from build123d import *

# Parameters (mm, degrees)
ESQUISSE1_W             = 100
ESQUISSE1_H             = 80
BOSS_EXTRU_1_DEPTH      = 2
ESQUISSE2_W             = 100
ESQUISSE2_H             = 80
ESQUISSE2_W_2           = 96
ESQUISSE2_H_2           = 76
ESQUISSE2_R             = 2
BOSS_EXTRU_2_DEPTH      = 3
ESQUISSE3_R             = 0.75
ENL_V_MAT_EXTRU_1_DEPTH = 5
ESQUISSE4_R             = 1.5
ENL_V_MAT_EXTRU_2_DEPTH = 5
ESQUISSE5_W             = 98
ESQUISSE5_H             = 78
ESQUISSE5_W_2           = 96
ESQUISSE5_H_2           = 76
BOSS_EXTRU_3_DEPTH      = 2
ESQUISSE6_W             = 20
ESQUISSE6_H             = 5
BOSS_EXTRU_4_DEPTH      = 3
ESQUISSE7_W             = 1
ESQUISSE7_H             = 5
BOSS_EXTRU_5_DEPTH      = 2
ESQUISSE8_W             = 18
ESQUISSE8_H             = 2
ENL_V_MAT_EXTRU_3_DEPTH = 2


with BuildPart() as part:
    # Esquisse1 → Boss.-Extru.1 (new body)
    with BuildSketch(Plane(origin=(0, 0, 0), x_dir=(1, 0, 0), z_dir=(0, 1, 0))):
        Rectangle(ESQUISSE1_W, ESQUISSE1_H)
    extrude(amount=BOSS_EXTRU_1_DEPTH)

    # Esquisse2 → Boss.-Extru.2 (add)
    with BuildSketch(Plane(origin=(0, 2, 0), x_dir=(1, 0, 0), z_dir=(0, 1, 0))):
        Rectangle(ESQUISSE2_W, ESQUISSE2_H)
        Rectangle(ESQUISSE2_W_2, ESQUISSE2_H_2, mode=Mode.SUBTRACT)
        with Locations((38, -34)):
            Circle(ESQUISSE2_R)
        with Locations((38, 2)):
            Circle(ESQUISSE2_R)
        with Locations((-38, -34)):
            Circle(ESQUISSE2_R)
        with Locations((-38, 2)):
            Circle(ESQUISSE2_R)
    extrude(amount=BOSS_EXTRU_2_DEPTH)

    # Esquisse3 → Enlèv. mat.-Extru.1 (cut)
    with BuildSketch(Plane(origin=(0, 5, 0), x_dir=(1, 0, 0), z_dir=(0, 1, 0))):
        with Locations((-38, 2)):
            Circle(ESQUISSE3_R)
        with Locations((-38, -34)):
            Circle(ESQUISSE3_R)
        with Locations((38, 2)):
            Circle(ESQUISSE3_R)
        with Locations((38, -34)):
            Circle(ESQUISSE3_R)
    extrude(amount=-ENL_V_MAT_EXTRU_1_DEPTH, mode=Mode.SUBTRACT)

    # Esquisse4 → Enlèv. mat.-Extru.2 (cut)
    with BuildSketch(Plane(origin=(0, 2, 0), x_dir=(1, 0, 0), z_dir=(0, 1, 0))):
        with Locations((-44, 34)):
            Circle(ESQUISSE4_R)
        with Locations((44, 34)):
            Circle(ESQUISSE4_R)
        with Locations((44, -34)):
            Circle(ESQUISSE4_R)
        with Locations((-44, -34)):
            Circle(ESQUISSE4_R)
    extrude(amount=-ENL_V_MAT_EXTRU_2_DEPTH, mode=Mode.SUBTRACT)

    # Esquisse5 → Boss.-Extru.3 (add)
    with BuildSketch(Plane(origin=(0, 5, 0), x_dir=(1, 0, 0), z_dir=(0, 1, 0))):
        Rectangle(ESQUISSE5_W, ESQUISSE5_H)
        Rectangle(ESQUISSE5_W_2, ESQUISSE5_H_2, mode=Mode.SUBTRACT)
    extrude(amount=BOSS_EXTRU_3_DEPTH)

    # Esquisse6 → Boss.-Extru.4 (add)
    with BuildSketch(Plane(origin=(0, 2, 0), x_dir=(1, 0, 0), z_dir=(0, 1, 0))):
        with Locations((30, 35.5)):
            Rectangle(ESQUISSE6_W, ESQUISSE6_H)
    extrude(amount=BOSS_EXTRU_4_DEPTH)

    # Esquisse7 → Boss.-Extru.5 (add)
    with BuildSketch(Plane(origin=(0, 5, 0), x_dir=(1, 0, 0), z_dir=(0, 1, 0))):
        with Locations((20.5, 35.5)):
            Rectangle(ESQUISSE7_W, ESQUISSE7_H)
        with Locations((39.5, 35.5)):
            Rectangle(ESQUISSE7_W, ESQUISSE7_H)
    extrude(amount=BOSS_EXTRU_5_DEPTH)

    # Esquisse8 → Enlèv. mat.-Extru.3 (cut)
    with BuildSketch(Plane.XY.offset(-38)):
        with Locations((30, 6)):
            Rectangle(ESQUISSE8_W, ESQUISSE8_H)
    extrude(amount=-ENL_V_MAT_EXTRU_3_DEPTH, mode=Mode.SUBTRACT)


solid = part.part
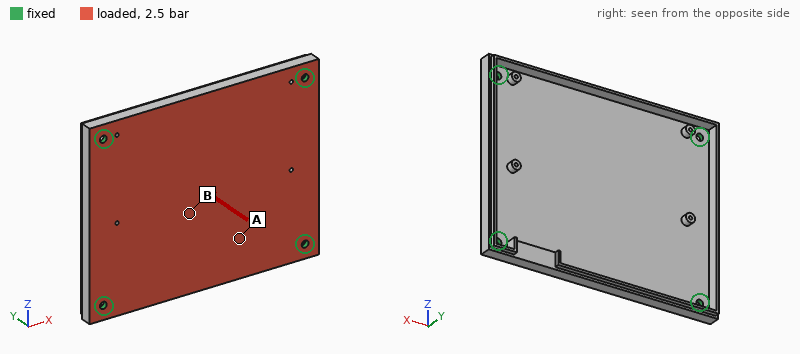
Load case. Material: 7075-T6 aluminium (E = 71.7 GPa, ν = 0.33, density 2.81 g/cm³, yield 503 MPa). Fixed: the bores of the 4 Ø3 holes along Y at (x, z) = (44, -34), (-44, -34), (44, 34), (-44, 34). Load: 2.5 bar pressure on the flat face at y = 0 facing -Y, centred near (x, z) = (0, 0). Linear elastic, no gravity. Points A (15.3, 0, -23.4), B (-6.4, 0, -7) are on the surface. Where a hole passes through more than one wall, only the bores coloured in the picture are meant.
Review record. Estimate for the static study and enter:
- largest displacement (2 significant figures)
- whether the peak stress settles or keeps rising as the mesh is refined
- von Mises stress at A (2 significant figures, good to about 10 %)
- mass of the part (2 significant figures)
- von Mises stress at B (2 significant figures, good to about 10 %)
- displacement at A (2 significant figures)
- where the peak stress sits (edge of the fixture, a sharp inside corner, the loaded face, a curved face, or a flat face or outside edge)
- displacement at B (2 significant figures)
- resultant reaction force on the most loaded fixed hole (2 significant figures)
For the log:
0.93 mm
keeps rising
49 MPa
54 g
110 MPa
0.54 mm
edge of the fixture
0.88 mm
540 N
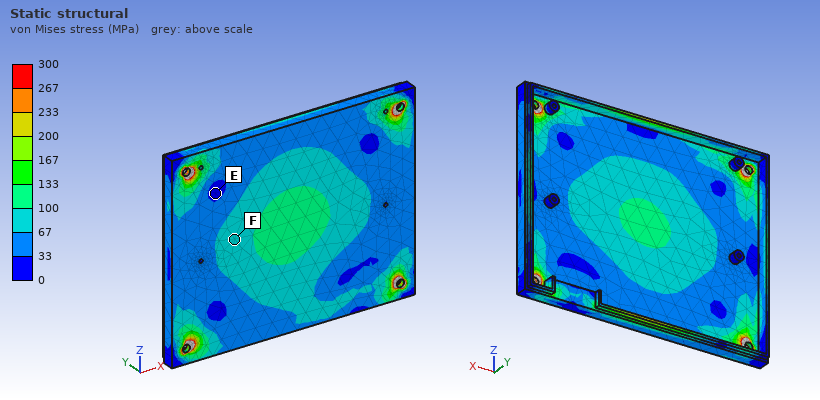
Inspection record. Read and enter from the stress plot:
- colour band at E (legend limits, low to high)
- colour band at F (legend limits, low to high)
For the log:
0 to 33 MPa
67 to 100 MPa
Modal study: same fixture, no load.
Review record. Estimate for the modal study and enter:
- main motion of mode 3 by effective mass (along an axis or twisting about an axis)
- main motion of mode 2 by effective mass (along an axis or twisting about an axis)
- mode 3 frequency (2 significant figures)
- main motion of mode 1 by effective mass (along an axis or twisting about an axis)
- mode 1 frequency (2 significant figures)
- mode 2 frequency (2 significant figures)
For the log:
twisting about Z
twisting about X
2800 Hz
along Y
1400 Hz
2400 Hz
